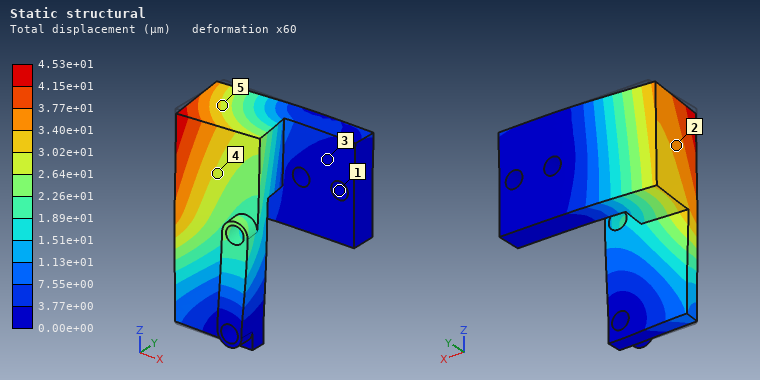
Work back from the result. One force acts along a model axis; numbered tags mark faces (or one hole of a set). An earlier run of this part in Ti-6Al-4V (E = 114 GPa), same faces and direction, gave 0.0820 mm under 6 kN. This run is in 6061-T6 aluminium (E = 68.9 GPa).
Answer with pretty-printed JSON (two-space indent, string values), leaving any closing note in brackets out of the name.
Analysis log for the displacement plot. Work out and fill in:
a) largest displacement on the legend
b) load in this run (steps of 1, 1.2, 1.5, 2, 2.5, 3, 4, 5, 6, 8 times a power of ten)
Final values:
{
  "largest displacement on the legend": "4.53e+01 µm",
  "load in this run": "2 kN"
}
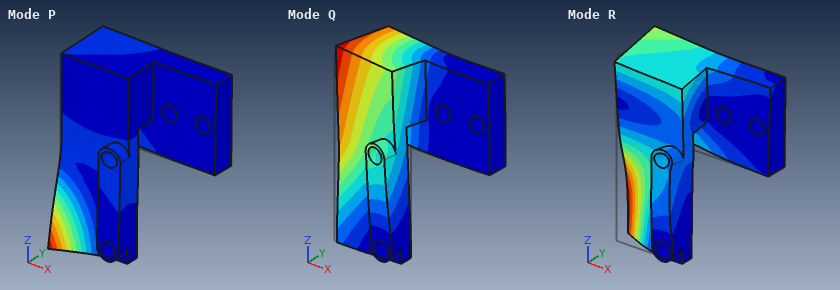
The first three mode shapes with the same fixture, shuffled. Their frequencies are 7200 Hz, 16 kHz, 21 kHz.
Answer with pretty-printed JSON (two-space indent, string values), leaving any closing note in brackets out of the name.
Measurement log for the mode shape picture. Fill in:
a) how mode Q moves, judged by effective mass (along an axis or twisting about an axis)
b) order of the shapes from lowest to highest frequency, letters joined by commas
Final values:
{
  "how mode Q moves, judged by effective mass": "along Y",
  "order of the shapes from lowest to highest frequency, letters joined by commas": "Q, R, P"
}
